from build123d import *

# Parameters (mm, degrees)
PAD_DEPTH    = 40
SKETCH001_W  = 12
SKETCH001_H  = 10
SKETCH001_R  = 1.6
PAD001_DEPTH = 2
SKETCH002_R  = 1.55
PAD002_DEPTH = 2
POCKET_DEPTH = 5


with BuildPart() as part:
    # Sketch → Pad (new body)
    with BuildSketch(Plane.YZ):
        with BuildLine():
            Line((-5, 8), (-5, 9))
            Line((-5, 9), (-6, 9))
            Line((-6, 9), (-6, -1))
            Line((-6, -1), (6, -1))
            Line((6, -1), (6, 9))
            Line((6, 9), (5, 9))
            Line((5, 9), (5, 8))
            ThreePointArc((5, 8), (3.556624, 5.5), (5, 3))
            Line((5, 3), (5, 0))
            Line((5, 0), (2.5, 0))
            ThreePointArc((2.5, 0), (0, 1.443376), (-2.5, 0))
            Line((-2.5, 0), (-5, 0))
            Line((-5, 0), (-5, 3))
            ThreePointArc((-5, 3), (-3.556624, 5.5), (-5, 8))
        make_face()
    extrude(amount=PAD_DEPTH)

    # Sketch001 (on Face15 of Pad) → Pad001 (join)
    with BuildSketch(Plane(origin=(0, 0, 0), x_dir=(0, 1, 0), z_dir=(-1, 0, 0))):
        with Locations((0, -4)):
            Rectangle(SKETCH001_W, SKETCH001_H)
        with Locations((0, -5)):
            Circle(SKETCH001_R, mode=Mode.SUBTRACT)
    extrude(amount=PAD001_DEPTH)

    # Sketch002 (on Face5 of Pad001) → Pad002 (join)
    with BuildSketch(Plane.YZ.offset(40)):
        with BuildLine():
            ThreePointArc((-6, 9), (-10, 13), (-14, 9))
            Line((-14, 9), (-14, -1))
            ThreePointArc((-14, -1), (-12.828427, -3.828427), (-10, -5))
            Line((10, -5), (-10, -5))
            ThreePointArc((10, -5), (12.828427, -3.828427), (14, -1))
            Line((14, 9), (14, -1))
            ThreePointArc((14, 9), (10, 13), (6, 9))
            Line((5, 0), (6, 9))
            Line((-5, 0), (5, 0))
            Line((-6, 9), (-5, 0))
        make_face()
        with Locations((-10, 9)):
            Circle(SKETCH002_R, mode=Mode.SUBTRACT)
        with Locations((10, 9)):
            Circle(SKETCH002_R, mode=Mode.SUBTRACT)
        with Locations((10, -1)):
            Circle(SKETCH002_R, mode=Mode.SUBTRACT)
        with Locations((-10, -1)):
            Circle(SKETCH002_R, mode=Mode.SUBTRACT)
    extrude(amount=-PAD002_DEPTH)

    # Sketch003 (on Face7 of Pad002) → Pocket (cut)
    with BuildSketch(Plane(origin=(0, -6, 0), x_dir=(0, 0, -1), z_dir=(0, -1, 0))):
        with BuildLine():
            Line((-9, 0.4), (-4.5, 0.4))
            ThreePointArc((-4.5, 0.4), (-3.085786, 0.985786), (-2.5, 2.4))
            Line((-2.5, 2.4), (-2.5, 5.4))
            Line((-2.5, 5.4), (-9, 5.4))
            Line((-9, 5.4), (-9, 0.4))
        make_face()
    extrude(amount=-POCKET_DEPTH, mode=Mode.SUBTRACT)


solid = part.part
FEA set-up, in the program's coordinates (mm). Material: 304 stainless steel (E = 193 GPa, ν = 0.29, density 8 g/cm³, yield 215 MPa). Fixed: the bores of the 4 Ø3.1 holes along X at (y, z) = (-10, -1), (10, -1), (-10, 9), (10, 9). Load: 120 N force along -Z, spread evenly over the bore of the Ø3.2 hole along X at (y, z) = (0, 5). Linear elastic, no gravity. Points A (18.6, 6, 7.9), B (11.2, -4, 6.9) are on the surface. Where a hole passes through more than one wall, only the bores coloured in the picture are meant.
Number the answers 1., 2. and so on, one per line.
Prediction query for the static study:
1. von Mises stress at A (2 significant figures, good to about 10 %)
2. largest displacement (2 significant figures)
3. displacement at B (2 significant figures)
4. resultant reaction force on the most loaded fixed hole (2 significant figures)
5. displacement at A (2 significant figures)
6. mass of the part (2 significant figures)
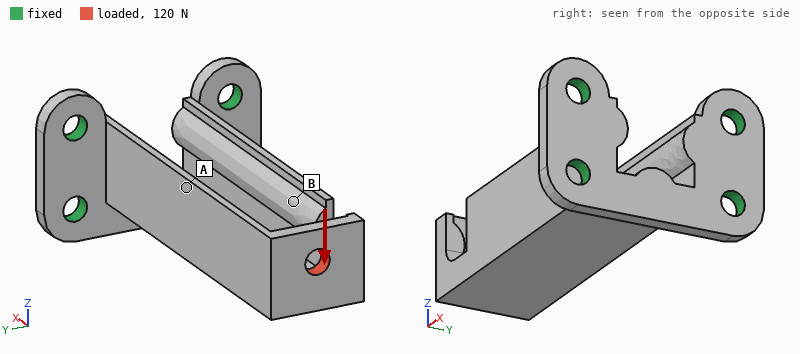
1. 32 MPa
2. 85 µm
3. 46 µm
4. 270 N
5. 36 µm
6. 20 g
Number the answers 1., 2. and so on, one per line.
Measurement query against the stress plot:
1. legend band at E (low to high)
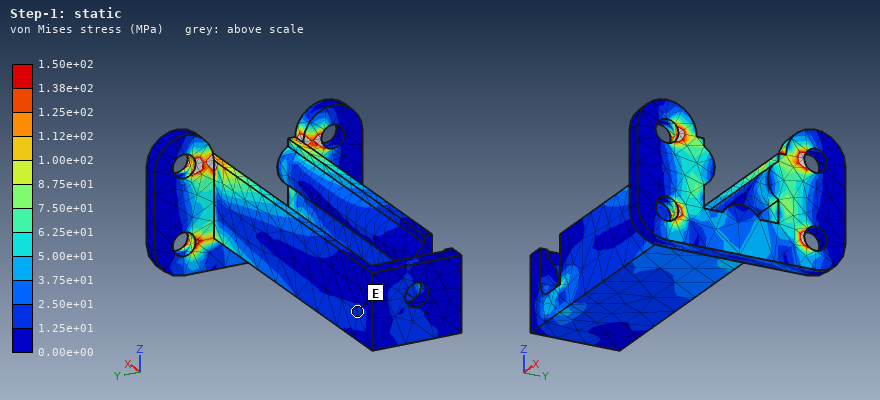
1. 1.25e+01 to 2.50e+01 MPa
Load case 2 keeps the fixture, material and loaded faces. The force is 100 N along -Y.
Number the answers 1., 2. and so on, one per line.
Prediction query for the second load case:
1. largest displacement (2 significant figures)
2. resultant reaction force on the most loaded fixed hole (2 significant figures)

1. 0.11 mm
2. 240 N
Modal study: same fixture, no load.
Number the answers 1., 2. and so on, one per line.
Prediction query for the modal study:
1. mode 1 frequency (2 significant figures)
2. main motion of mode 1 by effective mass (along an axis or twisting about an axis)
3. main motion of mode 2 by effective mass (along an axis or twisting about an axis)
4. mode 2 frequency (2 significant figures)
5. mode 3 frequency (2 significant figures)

1. 2500 Hz
2. along Y
3. along Z
4. 2700 Hz
5. 6300 Hz
